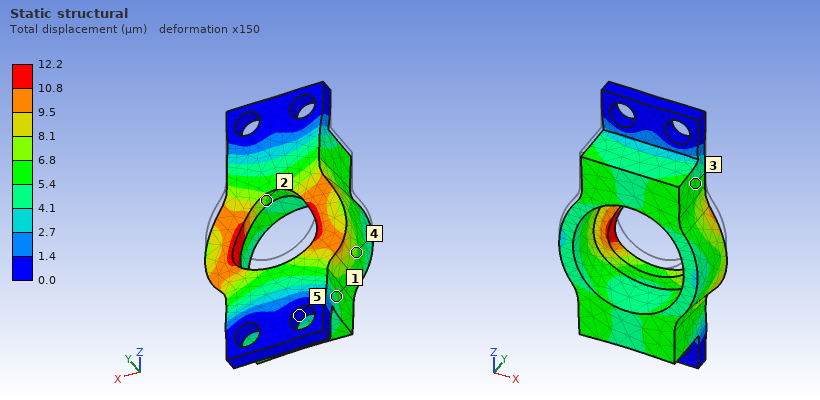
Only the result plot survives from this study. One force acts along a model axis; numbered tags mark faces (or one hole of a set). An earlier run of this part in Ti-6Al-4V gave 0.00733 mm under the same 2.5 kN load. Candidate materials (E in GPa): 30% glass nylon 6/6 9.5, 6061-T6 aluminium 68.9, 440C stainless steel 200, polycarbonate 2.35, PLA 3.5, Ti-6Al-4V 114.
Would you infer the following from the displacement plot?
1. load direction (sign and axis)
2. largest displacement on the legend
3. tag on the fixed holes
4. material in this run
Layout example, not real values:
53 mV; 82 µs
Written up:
-Z; 12.2 µm; 5; 6061-T6 aluminium
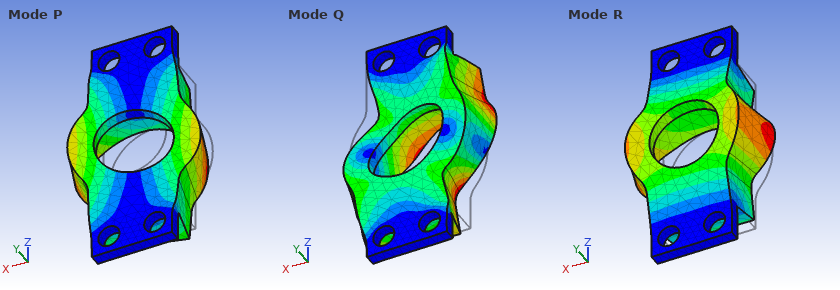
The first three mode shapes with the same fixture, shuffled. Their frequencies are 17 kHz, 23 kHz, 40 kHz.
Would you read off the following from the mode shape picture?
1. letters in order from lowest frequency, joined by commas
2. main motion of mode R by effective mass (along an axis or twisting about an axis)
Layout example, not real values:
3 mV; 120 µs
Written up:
R, P, Q; along Y
